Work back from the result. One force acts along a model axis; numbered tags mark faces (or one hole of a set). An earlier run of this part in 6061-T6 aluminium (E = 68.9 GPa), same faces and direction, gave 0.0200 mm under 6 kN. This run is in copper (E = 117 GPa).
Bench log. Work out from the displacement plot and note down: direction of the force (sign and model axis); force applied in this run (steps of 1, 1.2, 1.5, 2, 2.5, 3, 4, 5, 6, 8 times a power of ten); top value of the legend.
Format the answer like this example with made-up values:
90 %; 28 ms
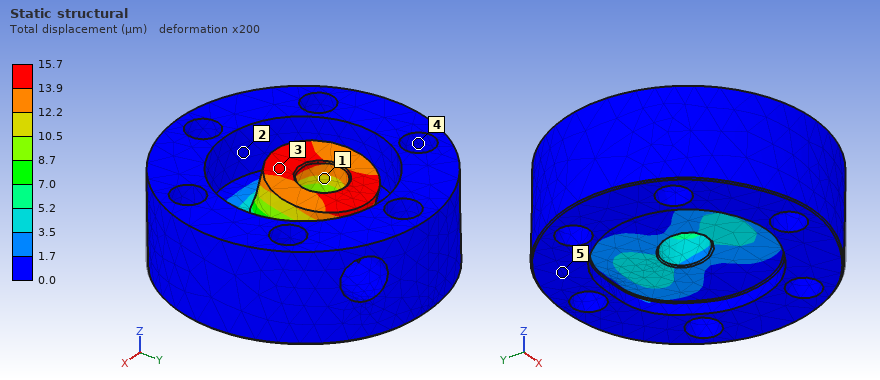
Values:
+Y; 8 kN; 15.7 µm
